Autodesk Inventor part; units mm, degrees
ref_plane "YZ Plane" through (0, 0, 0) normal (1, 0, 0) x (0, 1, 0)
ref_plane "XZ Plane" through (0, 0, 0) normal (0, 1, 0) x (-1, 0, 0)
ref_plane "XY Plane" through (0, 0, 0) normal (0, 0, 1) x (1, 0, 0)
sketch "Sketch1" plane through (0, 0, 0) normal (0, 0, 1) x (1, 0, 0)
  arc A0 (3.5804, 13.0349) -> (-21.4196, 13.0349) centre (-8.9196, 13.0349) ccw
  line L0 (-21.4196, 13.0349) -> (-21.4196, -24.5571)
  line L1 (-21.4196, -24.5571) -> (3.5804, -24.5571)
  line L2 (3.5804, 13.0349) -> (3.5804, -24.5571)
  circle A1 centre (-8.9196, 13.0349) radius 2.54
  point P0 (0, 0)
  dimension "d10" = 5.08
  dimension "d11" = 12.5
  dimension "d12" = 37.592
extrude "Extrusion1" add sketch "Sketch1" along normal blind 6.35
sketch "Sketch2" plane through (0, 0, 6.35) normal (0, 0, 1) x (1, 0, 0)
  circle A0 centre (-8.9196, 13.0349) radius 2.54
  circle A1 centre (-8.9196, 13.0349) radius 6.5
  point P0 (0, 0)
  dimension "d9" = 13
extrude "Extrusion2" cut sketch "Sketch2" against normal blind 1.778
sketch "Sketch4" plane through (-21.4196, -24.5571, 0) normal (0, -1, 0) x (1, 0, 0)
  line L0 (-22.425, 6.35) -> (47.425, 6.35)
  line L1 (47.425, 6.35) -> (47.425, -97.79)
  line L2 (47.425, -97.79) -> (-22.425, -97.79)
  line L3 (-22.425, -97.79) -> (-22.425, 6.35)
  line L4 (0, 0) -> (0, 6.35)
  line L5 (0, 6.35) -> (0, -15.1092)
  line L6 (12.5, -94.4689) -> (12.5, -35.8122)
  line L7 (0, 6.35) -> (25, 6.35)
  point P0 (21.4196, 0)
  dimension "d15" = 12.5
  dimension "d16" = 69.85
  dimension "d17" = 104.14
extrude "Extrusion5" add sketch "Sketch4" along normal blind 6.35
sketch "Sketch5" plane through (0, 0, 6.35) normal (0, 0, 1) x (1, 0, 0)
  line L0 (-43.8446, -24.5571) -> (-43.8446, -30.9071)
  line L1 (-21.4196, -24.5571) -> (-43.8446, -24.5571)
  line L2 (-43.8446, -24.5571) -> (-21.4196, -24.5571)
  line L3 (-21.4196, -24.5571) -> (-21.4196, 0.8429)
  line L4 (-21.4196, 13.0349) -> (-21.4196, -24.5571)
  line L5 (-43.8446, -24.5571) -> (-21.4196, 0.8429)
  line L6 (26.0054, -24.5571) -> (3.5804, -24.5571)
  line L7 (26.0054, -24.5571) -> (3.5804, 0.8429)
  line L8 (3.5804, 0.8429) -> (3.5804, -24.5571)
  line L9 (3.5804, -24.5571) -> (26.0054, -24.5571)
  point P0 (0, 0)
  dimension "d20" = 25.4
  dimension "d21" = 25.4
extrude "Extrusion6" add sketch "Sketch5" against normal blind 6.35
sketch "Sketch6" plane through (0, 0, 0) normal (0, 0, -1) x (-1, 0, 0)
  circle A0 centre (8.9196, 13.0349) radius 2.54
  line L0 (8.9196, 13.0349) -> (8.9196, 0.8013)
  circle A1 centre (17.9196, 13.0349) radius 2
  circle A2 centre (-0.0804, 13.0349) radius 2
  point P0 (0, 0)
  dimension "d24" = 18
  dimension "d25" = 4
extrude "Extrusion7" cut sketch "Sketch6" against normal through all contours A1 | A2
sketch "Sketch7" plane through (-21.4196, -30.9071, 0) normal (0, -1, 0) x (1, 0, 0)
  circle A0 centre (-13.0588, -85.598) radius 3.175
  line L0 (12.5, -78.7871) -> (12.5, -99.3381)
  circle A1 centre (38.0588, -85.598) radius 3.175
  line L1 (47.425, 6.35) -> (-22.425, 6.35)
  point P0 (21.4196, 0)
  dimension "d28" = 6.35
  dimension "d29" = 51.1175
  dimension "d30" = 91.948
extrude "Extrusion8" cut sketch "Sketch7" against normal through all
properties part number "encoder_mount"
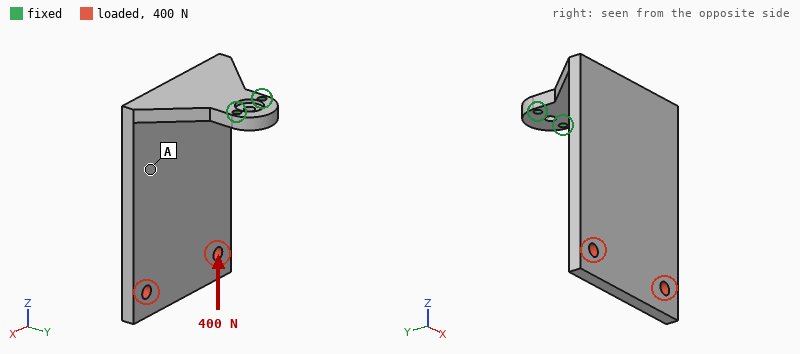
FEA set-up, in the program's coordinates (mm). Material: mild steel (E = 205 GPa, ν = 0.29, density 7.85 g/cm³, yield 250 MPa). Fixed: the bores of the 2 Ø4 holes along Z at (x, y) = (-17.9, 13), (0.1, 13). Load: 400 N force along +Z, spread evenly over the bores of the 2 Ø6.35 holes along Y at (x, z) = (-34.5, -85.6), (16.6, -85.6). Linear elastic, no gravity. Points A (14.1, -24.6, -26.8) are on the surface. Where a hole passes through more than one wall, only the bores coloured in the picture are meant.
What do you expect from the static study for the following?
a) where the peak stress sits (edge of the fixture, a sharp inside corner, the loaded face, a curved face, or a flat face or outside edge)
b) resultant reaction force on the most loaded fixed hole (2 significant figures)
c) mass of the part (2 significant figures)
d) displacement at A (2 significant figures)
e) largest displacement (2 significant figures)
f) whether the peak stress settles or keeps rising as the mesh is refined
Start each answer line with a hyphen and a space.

- edge of the fixture
- 210 N
- 440 g
- 0.11 mm
- 0.30 mm
- keeps rising
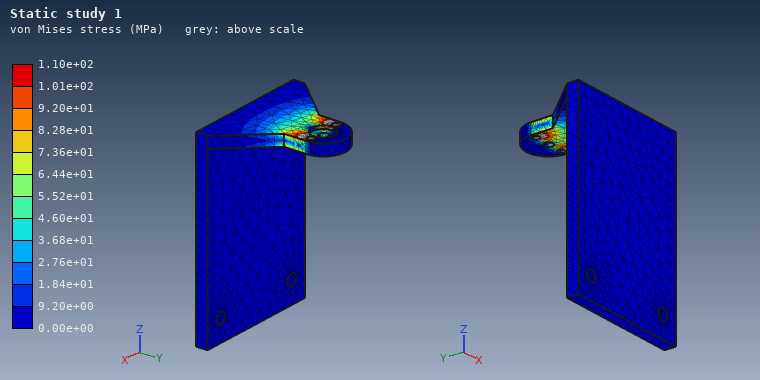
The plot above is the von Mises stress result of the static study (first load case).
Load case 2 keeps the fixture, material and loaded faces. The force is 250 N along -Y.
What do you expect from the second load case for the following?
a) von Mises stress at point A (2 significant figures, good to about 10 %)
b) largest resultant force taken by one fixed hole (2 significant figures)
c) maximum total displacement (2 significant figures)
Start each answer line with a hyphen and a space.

- 30 MPa
- 140 N
- 0.87 mm
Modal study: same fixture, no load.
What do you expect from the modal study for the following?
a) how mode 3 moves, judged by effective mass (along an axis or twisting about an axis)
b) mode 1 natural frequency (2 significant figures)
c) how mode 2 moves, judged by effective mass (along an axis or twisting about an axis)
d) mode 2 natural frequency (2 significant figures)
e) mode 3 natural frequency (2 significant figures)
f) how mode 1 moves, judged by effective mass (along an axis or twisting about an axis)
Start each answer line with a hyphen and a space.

- along Z
- 230 Hz
- along X
- 360 Hz
- 1000 Hz
- along Y
